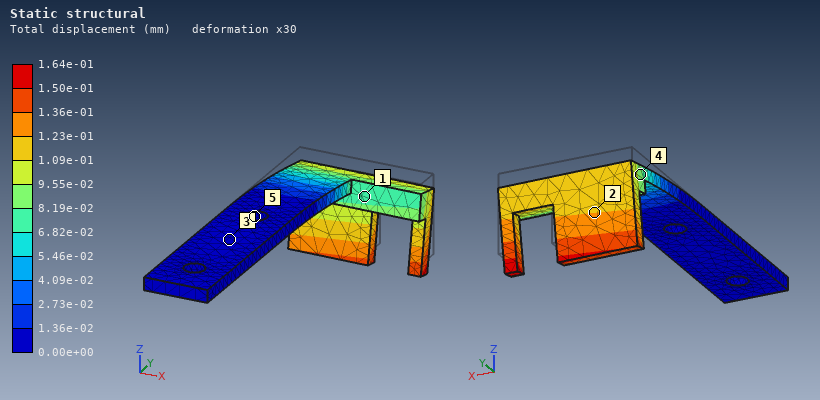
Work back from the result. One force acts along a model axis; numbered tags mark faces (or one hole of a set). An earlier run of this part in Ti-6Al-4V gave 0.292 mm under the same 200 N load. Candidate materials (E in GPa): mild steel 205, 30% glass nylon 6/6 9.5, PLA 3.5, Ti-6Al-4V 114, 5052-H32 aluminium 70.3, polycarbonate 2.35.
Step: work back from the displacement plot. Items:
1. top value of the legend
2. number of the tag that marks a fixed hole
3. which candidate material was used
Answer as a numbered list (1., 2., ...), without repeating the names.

1. 1.64e-01 mm
2. 5
3. mild steel
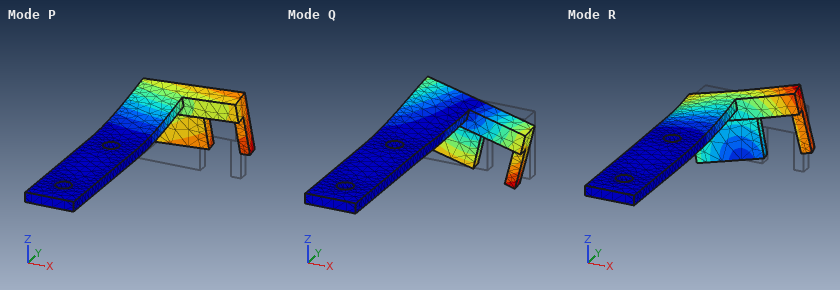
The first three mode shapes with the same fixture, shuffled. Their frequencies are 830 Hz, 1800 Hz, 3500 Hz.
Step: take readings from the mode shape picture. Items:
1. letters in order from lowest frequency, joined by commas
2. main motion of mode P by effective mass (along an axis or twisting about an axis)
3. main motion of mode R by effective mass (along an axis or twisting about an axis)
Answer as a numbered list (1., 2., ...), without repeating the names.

1. P, Q, R
2. along Z
3. along X
